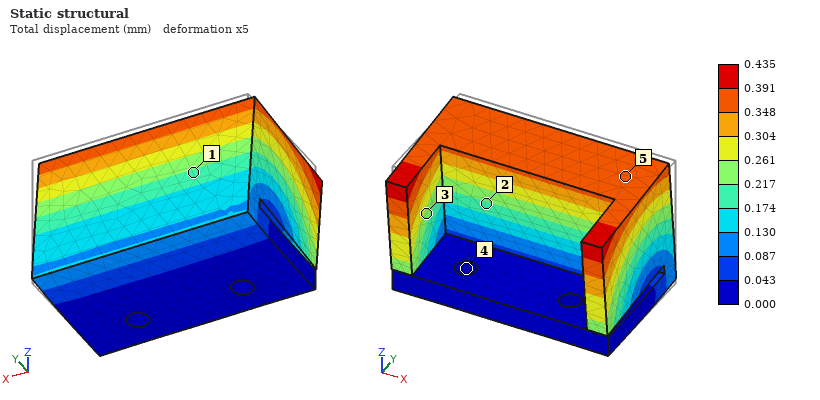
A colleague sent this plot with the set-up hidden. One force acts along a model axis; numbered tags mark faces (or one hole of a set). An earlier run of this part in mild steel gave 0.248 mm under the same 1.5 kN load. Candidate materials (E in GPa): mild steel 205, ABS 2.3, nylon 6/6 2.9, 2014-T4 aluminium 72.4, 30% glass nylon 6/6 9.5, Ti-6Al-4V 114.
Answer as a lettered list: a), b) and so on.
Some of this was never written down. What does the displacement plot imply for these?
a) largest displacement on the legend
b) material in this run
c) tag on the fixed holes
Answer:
a) 0.435 mm
b) Ti-6Al-4V
c) 4
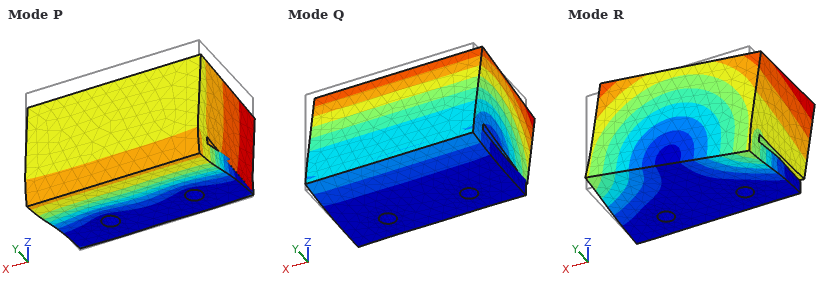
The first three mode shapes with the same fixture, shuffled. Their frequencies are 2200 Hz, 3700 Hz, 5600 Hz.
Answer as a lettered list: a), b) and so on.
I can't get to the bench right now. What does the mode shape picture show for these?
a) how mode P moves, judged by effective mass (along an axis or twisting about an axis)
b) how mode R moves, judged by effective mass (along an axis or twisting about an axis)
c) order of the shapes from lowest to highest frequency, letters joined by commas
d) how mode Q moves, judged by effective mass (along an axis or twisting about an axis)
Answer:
a) along Z
b) along X
c) Q, R, P
d) along Y
